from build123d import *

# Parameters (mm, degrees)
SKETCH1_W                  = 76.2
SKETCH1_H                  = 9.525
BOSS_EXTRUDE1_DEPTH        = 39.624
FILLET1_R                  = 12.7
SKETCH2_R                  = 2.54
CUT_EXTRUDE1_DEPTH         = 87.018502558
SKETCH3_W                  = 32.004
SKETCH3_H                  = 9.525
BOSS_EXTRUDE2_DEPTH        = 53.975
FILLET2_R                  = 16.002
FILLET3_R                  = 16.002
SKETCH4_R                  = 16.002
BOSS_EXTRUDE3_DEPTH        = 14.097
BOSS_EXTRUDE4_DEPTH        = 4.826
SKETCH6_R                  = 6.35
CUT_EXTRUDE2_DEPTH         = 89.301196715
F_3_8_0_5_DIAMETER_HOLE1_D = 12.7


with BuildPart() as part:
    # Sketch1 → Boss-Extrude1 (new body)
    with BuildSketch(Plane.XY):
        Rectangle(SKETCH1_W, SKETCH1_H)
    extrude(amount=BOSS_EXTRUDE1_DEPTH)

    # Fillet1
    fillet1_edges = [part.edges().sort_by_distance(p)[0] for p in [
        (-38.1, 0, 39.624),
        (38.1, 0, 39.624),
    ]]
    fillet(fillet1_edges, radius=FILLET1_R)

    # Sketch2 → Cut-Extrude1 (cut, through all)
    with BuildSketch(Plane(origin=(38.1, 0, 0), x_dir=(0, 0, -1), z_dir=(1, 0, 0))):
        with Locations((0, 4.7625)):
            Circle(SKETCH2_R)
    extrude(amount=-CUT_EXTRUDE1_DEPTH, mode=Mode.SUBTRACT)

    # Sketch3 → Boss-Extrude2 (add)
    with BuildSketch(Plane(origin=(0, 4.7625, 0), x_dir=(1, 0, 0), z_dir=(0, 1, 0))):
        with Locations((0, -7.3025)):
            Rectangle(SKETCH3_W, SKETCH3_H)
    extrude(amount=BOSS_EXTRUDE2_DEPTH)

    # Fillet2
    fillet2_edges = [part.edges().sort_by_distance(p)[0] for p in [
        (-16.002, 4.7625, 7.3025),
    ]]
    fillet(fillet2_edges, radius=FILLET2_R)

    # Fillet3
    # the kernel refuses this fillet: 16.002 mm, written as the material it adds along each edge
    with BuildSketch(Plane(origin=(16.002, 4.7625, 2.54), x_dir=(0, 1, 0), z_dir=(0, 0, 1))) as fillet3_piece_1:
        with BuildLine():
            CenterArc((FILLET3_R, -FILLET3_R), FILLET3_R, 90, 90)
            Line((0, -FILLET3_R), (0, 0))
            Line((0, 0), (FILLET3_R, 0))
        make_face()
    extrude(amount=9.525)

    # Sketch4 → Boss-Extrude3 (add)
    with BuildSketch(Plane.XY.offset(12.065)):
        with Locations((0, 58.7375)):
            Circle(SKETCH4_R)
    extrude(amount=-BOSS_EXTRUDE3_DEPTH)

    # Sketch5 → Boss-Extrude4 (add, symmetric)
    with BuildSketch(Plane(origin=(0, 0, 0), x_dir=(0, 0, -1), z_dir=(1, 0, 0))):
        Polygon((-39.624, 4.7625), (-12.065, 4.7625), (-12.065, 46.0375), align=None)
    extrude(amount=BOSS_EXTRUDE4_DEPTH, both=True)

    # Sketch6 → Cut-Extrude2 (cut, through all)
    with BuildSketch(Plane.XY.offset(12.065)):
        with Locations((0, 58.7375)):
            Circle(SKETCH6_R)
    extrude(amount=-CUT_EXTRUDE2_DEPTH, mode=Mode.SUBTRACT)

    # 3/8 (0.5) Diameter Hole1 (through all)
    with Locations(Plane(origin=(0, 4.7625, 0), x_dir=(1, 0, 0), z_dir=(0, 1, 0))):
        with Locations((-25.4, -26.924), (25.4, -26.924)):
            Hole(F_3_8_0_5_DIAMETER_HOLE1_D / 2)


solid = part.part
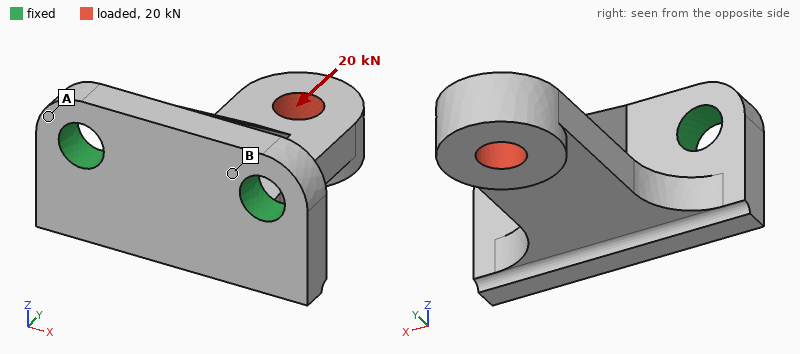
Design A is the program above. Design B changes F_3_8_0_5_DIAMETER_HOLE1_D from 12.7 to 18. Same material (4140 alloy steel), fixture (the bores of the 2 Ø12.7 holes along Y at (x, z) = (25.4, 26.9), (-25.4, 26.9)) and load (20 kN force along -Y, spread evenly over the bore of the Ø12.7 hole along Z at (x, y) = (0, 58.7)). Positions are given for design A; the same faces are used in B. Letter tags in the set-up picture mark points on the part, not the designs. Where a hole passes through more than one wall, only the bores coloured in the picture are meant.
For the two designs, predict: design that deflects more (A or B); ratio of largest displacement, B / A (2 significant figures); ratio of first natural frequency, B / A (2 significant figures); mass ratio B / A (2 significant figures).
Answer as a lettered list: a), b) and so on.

a) A
b) 0.77
c) 1.1
d) 0.95
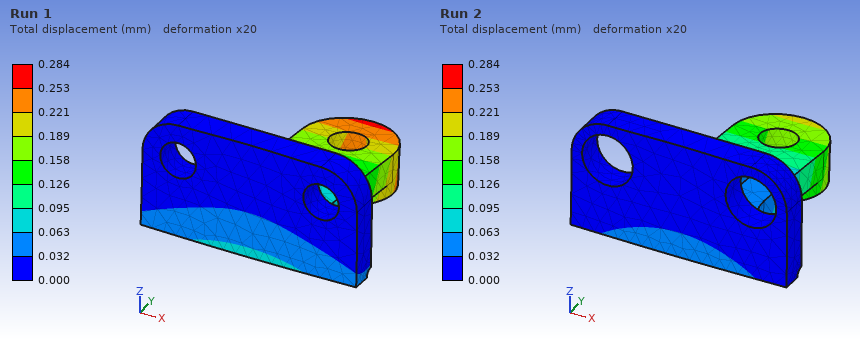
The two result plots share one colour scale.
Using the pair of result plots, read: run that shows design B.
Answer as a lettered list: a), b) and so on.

a) Run 2
